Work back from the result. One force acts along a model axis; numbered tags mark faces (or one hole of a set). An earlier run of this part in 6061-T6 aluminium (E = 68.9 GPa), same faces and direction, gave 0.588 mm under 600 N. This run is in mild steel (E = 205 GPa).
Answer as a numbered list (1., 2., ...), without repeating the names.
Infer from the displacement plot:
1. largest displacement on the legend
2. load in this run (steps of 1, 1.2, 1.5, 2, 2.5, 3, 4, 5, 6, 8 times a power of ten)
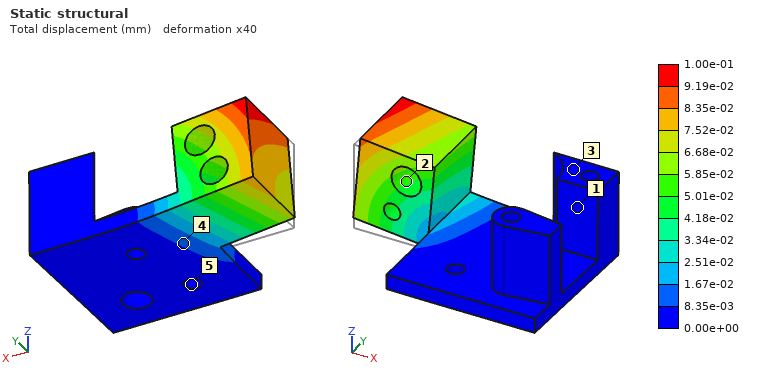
1. 1.00e-01 mm
2. 300 N
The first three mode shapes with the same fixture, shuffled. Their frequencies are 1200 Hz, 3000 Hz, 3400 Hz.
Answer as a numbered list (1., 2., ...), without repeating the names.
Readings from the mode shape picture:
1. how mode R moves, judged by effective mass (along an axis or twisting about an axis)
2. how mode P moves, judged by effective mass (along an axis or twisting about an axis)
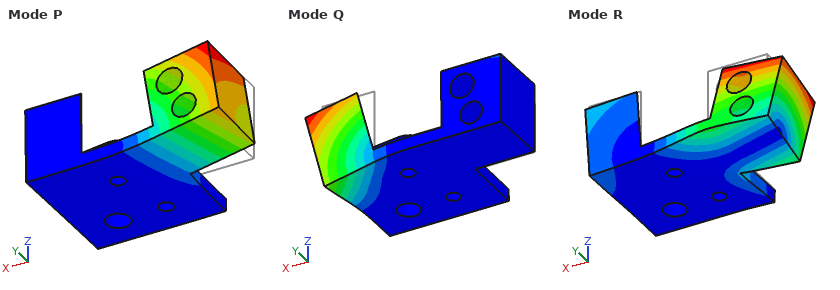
1. along Y
2. along Z
